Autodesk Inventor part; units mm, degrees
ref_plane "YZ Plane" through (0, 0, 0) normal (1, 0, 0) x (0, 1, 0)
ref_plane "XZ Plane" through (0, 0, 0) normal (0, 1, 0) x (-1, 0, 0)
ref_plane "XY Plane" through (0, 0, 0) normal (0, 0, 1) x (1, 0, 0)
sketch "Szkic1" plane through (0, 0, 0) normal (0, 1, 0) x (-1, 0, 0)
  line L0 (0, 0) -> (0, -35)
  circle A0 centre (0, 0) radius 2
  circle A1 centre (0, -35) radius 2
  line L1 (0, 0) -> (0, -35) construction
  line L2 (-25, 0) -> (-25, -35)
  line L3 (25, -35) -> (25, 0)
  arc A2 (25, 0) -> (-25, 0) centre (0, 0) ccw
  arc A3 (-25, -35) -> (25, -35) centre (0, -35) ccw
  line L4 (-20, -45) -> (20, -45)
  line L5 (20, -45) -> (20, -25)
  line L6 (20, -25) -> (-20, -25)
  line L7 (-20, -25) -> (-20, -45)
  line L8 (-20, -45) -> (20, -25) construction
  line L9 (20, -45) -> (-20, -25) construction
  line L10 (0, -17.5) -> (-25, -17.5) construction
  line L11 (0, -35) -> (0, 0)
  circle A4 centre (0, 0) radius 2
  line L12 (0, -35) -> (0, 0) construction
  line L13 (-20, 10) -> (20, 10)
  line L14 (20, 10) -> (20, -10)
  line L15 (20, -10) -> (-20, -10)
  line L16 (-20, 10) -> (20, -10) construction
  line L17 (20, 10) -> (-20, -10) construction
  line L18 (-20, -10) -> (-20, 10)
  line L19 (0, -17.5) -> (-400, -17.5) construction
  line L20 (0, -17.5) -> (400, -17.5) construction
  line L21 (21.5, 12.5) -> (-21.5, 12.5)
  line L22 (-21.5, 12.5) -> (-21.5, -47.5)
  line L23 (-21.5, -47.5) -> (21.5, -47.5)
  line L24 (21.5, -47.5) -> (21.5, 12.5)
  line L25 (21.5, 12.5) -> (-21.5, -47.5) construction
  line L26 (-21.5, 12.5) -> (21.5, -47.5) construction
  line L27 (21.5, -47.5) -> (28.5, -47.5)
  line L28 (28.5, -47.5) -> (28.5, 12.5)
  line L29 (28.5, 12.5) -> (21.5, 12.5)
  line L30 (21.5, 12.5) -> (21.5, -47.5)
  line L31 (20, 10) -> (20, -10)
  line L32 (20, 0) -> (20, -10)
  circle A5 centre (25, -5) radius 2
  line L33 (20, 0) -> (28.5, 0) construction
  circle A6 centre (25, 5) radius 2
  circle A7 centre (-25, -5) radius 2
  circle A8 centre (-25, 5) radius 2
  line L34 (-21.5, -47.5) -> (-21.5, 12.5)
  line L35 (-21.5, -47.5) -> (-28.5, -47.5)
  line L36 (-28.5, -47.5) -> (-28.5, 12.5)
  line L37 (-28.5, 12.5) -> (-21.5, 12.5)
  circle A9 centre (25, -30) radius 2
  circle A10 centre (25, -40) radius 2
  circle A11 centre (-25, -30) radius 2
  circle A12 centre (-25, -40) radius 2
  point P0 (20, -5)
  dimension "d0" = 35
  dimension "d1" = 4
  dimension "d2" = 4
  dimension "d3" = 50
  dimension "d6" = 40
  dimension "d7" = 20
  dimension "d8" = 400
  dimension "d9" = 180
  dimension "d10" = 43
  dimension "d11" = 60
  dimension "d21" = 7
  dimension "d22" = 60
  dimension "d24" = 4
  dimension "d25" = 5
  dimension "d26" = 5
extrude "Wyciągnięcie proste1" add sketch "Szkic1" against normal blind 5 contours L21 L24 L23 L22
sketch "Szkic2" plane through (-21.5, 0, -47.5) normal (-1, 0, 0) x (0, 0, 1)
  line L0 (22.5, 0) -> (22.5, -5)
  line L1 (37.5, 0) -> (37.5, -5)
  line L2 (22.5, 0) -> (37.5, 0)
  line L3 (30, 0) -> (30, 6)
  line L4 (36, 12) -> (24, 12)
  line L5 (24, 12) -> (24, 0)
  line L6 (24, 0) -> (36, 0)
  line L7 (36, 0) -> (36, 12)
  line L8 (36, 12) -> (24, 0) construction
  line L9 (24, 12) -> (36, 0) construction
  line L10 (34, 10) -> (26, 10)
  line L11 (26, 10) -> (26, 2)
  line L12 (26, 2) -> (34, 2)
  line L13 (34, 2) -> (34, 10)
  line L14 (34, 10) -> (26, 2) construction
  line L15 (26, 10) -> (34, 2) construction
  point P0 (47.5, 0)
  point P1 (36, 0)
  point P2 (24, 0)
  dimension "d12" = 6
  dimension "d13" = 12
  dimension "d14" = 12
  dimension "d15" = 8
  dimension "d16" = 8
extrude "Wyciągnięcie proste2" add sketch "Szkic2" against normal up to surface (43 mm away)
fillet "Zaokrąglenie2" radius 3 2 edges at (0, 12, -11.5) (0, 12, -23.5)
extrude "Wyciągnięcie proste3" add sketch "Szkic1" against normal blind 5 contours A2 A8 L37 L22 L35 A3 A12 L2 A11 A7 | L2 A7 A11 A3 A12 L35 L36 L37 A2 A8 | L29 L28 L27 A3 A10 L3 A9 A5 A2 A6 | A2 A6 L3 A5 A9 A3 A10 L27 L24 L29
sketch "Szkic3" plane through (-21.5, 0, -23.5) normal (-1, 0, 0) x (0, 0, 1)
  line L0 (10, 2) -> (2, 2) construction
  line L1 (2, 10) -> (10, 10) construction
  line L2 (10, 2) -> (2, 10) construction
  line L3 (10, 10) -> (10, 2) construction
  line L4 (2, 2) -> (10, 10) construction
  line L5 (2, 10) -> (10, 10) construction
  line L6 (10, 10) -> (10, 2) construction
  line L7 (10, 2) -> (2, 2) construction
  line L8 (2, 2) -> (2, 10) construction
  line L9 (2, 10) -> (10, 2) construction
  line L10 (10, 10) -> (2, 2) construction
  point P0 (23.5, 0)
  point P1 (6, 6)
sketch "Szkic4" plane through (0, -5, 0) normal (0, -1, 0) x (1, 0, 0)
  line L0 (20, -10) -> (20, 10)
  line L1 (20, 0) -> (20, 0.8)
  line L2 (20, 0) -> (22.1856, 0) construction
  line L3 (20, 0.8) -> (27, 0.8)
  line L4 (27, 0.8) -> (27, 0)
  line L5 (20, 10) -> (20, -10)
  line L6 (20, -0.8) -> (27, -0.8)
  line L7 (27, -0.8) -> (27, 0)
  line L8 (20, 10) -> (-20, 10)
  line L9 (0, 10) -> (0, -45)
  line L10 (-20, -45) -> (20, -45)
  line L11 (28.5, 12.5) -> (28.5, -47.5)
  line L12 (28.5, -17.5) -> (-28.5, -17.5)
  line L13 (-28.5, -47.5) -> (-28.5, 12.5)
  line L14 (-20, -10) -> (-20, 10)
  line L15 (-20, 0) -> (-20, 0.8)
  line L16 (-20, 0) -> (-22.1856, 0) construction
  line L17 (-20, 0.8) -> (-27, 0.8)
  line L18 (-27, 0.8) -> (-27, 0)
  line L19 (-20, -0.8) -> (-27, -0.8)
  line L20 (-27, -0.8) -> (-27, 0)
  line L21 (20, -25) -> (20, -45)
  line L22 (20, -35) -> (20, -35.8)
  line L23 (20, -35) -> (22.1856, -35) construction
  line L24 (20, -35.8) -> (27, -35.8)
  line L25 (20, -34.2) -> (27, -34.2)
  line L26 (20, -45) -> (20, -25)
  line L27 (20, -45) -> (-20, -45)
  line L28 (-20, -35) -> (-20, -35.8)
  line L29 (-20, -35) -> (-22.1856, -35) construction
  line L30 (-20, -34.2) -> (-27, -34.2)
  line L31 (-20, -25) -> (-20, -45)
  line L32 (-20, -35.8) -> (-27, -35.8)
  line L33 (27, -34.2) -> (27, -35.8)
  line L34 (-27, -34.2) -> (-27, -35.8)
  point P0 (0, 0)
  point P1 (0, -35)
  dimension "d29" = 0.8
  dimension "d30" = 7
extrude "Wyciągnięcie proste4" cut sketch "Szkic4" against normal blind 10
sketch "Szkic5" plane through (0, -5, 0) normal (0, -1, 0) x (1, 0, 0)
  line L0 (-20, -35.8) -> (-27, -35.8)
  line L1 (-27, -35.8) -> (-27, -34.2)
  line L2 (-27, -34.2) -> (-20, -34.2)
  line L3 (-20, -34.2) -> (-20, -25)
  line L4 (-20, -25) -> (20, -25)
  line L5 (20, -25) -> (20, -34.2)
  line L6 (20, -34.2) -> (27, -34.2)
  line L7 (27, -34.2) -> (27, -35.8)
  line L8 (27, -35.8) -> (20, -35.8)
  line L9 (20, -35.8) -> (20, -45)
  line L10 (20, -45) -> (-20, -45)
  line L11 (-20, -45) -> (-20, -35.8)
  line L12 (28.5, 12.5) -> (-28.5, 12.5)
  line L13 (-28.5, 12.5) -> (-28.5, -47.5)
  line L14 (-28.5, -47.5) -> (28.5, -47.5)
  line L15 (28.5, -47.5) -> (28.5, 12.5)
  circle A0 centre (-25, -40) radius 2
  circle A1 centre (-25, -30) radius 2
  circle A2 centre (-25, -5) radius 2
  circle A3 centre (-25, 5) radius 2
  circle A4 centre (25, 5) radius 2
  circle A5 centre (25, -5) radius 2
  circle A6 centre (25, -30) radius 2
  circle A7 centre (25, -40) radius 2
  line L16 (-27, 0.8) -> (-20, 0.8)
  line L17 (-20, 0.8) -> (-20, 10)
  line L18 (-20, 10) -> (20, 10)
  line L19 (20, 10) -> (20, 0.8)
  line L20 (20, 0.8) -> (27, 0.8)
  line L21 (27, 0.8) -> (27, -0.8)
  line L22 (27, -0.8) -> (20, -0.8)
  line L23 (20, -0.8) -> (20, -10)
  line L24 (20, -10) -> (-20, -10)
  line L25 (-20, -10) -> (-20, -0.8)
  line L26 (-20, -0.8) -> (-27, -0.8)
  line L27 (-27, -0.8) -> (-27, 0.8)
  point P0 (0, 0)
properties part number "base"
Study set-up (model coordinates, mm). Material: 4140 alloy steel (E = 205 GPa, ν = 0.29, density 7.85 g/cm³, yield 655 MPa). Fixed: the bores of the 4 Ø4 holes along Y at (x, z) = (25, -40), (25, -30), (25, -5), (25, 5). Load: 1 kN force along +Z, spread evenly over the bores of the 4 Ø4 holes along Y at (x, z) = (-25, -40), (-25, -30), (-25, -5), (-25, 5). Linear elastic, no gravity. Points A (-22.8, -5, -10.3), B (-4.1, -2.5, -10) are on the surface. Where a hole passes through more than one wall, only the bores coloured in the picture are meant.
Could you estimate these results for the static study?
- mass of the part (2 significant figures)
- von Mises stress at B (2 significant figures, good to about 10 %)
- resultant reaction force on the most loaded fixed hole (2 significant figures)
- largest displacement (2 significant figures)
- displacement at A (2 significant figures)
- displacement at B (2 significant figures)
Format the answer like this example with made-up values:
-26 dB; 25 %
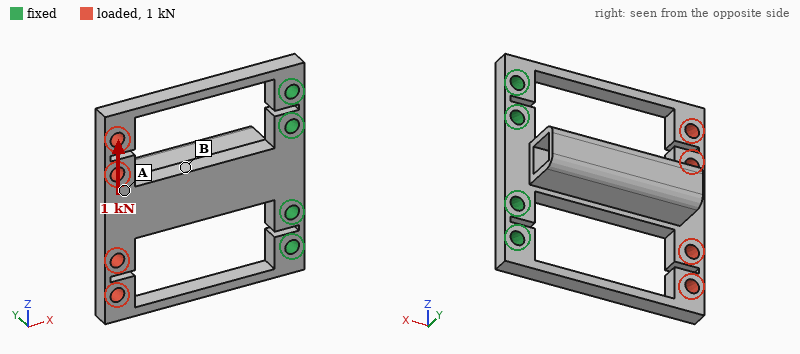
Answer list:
91 g; 49 MPa; 2.1 kN; 0.14 mm; 0.098 mm; 0.049 mm
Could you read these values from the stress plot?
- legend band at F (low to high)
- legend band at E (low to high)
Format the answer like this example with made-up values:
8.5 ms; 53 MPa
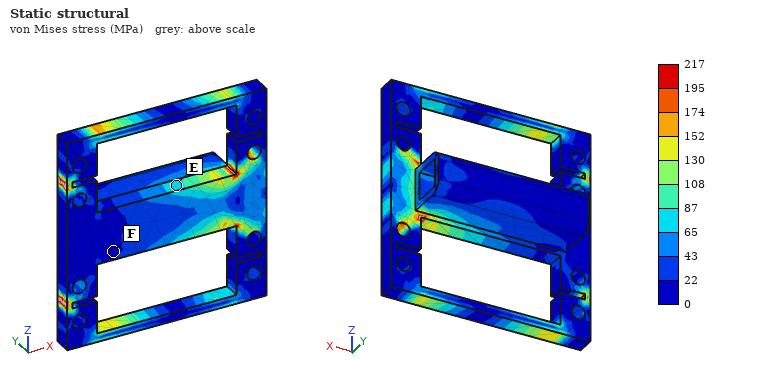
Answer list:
0 to 22 MPa; 65 to 87 MPa
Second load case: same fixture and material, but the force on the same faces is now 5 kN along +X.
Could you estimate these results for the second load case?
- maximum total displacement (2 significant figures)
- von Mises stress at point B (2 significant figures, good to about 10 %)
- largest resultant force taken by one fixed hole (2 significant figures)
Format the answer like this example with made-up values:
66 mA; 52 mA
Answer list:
65 µm; 39 MPa; 2.0 kN
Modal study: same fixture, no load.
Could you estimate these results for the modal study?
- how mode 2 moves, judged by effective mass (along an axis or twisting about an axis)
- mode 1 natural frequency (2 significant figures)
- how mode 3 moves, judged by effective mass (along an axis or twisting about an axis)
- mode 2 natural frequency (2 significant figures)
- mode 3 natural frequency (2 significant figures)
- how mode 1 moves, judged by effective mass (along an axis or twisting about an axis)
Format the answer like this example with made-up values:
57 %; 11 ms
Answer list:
along Z; 1100 Hz; twisting about X; 2600 Hz; 3100 Hz; along Y
